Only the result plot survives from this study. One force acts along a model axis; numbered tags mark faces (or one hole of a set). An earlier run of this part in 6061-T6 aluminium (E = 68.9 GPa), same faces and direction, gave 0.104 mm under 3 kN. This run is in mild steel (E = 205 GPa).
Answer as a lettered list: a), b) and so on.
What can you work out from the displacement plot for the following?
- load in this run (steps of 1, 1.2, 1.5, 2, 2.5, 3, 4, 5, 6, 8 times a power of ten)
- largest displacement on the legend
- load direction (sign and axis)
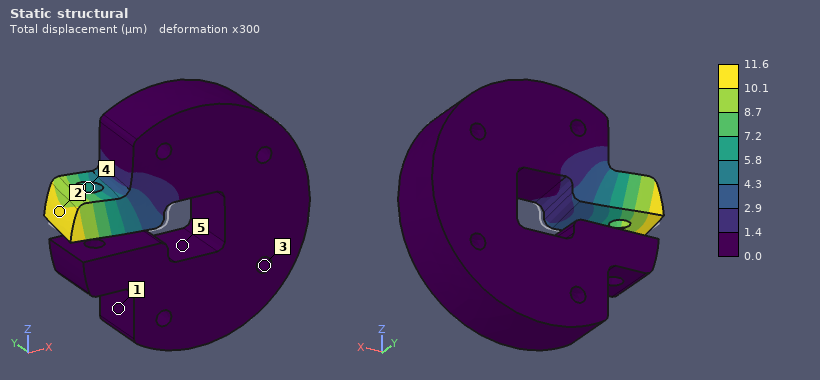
a) 1 kN
b) 11.6 µm
c) +Y
